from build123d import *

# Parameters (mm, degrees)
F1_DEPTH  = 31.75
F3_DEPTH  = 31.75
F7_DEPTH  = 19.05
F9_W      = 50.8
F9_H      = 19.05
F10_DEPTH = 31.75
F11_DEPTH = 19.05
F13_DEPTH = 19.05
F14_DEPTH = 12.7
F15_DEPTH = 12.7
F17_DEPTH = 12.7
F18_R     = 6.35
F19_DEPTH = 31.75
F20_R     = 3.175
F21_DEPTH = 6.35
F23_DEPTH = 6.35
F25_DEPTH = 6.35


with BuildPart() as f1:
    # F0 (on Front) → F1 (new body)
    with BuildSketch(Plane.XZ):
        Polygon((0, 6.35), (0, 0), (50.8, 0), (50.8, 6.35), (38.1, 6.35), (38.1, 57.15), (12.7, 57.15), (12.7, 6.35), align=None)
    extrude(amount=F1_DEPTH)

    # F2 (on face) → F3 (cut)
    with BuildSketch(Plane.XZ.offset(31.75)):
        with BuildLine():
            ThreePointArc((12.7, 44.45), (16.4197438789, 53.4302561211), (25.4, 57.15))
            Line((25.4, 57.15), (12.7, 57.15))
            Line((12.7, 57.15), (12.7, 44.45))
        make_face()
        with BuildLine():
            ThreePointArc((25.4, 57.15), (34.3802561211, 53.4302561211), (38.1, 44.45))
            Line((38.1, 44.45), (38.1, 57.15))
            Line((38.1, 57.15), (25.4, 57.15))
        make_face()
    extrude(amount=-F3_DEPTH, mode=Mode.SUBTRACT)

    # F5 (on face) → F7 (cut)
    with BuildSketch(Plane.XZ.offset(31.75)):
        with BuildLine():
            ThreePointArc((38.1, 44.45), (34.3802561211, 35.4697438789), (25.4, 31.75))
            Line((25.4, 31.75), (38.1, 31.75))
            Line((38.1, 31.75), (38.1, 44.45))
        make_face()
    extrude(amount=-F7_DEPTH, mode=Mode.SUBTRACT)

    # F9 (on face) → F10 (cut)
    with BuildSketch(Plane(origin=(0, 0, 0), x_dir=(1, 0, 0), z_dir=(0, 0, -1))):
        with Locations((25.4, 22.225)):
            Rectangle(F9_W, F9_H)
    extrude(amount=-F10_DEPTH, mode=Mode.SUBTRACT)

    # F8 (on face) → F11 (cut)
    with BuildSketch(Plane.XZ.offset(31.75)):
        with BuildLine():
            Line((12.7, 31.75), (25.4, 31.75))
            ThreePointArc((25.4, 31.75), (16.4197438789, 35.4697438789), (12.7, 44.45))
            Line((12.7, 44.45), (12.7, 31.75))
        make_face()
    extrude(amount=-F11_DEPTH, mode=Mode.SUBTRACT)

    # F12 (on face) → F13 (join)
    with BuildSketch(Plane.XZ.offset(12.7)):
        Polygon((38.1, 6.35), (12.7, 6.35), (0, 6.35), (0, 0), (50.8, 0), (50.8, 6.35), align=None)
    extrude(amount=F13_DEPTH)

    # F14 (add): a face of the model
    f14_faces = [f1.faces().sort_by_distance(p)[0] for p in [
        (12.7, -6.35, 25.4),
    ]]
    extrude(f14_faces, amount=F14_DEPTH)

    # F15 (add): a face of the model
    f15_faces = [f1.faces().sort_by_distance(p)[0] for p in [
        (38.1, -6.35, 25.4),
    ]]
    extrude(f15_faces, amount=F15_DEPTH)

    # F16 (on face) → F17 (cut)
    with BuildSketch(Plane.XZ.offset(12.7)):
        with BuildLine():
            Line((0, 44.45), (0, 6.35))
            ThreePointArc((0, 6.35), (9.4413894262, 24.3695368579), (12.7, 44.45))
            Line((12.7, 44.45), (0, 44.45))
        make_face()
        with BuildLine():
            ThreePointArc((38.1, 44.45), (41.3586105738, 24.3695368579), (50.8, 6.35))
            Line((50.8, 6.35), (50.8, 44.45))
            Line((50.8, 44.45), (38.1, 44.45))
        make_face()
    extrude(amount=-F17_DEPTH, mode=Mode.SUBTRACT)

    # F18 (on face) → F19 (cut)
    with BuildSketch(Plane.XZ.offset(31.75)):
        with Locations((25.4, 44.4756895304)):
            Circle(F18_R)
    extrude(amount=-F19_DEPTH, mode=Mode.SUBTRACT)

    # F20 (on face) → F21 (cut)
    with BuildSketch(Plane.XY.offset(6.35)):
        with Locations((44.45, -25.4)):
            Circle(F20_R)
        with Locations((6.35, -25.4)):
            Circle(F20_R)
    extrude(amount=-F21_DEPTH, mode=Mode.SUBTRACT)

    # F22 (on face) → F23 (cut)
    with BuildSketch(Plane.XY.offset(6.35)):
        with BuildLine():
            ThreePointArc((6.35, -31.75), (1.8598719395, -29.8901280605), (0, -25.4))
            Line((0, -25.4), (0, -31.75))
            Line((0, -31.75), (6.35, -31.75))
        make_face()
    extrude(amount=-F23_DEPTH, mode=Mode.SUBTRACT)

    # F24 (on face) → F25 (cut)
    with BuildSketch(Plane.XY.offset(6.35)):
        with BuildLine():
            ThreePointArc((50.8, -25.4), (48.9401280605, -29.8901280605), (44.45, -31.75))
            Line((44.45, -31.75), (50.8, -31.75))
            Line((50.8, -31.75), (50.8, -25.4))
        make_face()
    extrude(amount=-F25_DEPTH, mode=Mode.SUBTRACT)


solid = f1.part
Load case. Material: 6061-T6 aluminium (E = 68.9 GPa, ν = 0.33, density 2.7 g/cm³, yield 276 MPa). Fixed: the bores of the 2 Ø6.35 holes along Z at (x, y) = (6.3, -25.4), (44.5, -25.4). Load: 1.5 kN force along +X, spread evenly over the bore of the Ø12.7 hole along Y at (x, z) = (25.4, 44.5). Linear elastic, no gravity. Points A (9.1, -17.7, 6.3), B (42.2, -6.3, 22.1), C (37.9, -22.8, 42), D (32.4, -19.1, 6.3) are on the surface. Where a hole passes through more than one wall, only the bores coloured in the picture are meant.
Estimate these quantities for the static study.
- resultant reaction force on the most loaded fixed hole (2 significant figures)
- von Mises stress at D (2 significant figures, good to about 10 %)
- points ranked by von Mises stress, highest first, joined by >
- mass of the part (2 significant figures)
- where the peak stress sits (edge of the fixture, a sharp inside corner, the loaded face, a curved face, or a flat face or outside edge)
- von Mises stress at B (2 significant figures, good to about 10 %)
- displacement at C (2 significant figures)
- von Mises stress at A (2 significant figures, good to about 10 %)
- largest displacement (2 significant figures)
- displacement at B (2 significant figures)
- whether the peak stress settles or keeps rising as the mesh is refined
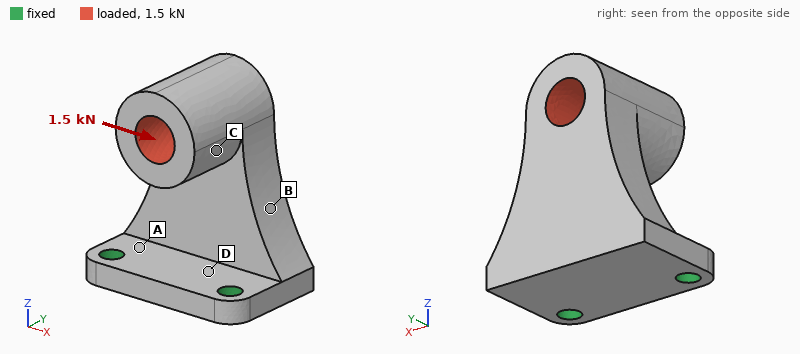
1.8 kN
36 MPa
A > D > B > C
94 g
edge of the fixture
20 MPa
0.11 mm
46 MPa
0.16 mm
0.052 mm
keeps rising
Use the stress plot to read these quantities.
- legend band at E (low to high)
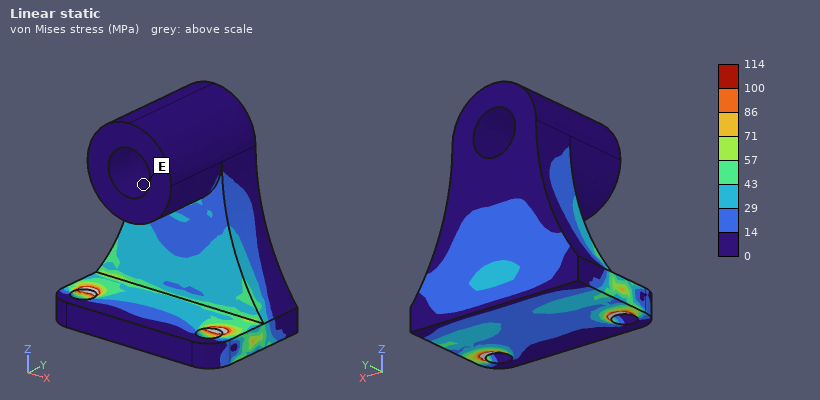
0 to 14 MPa
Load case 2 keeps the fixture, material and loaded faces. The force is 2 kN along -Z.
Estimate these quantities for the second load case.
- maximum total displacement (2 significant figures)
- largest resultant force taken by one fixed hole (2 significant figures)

54 µm
1.0 kN
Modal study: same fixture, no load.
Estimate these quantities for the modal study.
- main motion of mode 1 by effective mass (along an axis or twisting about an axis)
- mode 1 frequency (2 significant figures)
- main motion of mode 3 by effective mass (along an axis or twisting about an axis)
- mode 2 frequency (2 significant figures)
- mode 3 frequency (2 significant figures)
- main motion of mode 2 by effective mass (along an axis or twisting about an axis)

along Y
1200 Hz
along Z
3000 Hz
4900 Hz
along X
